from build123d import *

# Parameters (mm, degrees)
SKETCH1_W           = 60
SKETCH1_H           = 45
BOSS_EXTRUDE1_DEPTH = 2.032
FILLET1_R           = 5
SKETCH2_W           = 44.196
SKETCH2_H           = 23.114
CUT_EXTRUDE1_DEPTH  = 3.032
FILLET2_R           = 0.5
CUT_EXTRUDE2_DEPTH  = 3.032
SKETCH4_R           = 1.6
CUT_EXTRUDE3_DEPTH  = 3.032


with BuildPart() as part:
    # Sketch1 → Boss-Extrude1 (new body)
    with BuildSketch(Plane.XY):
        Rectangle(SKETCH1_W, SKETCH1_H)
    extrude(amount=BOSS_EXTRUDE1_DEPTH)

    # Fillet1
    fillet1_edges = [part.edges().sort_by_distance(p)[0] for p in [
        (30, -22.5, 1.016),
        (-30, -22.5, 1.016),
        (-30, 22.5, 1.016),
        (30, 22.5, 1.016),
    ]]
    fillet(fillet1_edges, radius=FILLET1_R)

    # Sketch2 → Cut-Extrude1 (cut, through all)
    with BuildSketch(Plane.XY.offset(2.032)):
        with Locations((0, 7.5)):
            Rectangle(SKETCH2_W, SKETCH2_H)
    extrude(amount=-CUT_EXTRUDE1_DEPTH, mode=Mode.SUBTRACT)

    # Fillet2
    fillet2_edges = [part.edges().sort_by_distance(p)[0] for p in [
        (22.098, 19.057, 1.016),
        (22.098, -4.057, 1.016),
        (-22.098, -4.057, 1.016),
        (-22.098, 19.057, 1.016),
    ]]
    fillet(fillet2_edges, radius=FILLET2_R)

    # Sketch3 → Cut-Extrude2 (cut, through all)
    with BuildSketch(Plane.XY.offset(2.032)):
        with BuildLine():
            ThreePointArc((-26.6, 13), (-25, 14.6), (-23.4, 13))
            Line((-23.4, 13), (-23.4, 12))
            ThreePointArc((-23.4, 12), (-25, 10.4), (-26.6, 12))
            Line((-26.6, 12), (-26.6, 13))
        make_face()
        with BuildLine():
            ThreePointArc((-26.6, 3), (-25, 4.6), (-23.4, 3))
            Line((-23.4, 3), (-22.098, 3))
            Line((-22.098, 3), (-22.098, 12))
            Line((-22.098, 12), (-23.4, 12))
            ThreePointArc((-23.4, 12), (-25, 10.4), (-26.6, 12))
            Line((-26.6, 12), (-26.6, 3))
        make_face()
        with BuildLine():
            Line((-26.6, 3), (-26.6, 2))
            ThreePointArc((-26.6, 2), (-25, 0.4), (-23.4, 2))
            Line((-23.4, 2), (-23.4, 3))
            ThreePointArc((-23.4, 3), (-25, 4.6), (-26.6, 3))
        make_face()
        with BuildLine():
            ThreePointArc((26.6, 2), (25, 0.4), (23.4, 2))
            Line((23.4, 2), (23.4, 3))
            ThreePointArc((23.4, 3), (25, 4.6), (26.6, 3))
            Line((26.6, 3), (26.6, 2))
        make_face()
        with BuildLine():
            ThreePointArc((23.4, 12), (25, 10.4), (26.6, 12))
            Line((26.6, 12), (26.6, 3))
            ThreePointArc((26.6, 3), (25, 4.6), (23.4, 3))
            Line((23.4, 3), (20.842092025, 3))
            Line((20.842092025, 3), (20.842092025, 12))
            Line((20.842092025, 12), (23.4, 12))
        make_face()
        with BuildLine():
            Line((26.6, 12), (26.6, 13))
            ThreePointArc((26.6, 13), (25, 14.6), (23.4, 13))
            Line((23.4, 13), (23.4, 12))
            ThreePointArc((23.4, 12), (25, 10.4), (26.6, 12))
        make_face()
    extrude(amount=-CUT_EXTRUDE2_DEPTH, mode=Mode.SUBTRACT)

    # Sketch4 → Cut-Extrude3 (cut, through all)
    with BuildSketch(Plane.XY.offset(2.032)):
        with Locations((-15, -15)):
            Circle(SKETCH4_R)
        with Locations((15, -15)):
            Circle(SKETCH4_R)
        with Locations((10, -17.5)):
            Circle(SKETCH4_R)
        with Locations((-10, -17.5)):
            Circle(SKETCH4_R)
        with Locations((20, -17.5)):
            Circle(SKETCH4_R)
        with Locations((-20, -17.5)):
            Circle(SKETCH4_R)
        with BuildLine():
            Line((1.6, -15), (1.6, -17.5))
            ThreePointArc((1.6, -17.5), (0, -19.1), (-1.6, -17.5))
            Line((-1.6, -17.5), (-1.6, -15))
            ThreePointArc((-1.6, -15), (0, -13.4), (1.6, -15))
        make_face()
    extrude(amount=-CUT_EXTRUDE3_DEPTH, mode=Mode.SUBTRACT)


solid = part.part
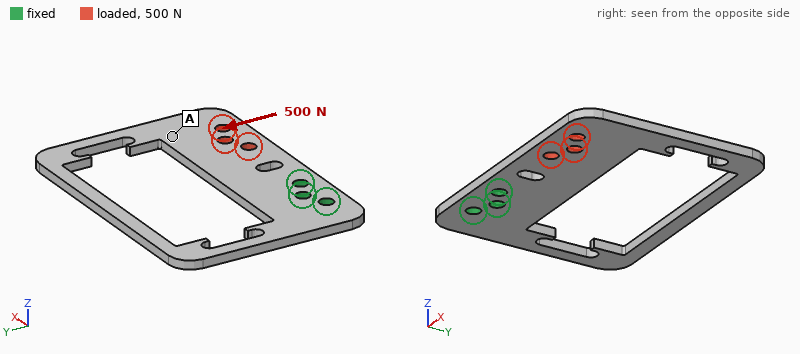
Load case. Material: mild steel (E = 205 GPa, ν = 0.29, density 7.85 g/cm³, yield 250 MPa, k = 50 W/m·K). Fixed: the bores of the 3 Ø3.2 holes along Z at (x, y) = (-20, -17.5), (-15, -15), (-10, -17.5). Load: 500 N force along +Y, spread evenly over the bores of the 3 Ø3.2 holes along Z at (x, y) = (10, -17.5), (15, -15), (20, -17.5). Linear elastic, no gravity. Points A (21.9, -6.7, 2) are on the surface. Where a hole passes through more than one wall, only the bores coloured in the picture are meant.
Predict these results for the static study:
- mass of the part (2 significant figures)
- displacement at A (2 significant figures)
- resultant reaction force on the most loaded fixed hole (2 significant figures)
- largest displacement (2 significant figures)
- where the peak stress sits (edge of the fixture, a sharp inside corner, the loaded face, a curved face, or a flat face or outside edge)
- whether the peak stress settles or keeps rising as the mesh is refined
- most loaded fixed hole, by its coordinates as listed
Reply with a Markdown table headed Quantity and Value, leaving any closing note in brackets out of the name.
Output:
| Quantity | Value |
|---|---|
| mass of the part | 24 g |
| displacement at A | 41 µm |
| resultant reaction force on the most loaded fixed hole | 1.4 kN |
| largest displacement | 55 µm |
| where the peak stress sits | edge of the fixture |
| whether the peak stress settles or keeps rising as the mesh is refined | keeps rising |
| most loaded fixed hole, by its coordinates as listed | (-10, -17.5) |
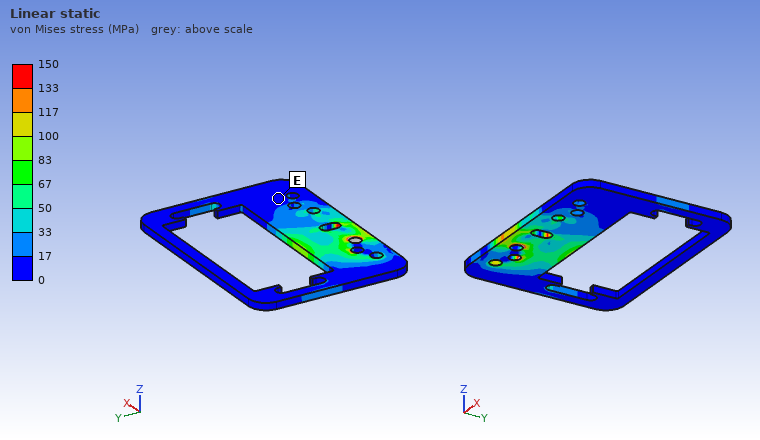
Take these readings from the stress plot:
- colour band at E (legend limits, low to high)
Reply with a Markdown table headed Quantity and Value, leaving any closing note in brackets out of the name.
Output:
| Quantity | Value |
|---|---|
| colour band at E | 0 to 17 MPa |
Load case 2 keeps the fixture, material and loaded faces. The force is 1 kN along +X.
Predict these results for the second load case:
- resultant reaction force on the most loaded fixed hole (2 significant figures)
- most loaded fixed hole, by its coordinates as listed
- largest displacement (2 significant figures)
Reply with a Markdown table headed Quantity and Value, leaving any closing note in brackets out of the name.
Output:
| Quantity | Value |
|---|---|
| resultant reaction force on the most loaded fixed hole | 710 N |
| most loaded fixed hole, by its coordinates as listed | (-10, -17.5) |
| largest displacement | 14 µm |
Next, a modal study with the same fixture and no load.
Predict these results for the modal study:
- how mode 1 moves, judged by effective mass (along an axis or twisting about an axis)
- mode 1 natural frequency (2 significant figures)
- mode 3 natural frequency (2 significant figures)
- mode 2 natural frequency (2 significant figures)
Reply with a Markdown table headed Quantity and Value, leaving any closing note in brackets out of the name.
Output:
| Quantity | Value |
|---|---|
| how mode 1 moves, judged by effective mass | along Z |
| mode 1 natural frequency | 610 Hz |
| mode 3 natural frequency | 1700 Hz |
| mode 2 natural frequency | 1000 Hz |
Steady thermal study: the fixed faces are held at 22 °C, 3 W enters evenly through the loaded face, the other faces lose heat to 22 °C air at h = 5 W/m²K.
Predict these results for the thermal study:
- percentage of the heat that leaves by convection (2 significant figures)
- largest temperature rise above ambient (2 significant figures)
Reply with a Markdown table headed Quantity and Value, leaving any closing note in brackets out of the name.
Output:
| Quantity | Value |
|---|---|
| percentage of the heat that leaves by convection | 12 % |
| largest temperature rise above ambient | 45 K |
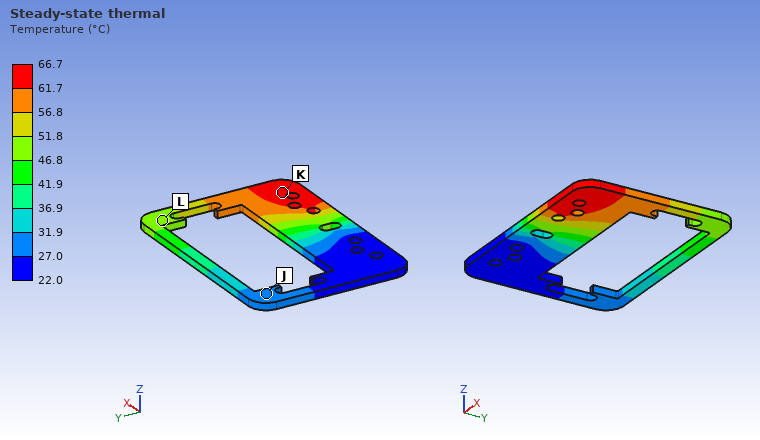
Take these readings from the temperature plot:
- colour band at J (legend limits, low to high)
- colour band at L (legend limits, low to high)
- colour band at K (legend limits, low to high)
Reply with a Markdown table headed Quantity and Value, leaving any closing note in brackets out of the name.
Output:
| Quantity | Value |
|---|---|
| colour band at J | 27.0 to 31.9 °C |
| colour band at L | 46.8 to 51.8 °C |
| colour band at K | 61.7 to 66.7 °C |
